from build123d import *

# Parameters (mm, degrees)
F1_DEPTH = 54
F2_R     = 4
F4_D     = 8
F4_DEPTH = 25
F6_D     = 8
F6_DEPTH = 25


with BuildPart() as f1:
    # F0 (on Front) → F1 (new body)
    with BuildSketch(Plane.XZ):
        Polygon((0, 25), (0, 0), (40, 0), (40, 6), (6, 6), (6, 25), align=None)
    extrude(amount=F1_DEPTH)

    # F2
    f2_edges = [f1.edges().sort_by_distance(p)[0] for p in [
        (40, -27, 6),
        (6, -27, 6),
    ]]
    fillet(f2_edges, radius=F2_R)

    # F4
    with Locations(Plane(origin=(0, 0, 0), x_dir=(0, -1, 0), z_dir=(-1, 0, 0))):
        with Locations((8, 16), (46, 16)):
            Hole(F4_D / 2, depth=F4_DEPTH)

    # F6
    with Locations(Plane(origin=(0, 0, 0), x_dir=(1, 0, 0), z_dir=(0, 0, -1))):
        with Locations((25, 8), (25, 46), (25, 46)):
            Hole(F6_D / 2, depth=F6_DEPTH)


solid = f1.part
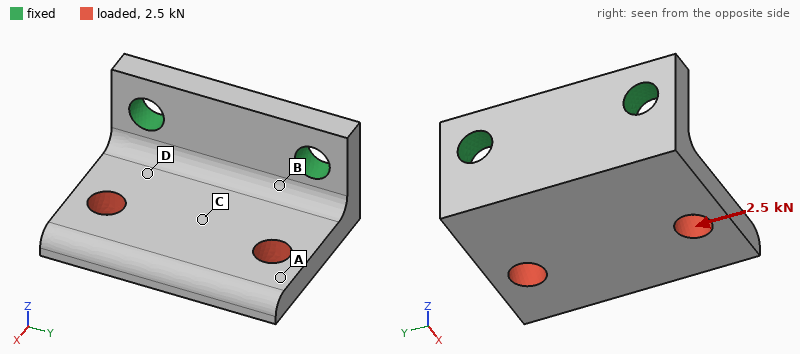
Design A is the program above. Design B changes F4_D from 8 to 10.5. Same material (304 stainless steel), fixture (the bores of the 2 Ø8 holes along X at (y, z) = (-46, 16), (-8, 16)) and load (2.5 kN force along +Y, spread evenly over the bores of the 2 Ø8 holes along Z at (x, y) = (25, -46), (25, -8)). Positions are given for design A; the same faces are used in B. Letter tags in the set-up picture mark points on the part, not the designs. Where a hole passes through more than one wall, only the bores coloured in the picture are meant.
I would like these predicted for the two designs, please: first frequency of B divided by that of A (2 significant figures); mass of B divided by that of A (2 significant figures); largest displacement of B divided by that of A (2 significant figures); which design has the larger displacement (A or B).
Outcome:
1.1
0.98
0.80
A
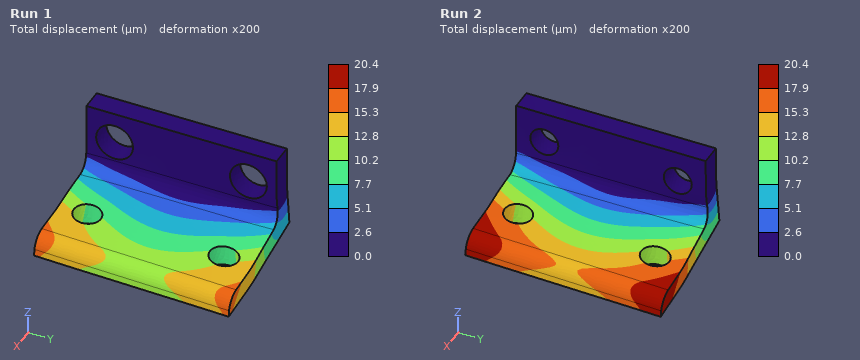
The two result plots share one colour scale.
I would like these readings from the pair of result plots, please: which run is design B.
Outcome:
Run 1
